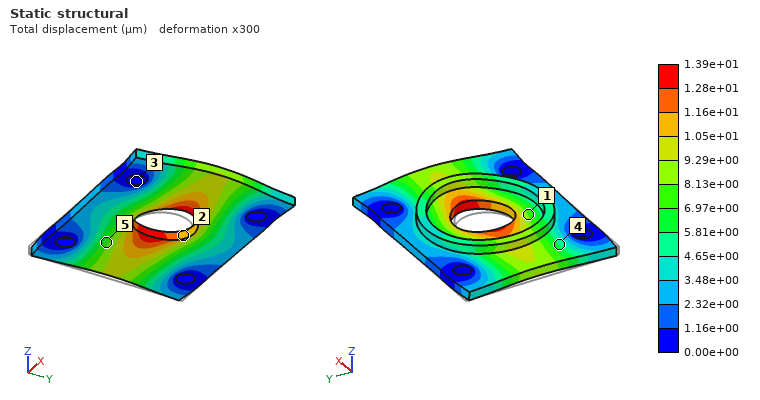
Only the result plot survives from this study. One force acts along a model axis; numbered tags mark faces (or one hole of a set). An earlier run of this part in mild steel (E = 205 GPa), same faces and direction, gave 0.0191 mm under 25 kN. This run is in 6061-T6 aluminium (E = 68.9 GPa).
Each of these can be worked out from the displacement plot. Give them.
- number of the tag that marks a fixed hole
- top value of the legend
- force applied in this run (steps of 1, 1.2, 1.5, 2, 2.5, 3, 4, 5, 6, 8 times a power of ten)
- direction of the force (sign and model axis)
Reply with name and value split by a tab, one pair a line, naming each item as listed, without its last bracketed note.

number of the tag that marks a fixed hole	3
top value of the legend	1.39e+01 µm
force applied in this run	6 kN
direction of the force	+X
